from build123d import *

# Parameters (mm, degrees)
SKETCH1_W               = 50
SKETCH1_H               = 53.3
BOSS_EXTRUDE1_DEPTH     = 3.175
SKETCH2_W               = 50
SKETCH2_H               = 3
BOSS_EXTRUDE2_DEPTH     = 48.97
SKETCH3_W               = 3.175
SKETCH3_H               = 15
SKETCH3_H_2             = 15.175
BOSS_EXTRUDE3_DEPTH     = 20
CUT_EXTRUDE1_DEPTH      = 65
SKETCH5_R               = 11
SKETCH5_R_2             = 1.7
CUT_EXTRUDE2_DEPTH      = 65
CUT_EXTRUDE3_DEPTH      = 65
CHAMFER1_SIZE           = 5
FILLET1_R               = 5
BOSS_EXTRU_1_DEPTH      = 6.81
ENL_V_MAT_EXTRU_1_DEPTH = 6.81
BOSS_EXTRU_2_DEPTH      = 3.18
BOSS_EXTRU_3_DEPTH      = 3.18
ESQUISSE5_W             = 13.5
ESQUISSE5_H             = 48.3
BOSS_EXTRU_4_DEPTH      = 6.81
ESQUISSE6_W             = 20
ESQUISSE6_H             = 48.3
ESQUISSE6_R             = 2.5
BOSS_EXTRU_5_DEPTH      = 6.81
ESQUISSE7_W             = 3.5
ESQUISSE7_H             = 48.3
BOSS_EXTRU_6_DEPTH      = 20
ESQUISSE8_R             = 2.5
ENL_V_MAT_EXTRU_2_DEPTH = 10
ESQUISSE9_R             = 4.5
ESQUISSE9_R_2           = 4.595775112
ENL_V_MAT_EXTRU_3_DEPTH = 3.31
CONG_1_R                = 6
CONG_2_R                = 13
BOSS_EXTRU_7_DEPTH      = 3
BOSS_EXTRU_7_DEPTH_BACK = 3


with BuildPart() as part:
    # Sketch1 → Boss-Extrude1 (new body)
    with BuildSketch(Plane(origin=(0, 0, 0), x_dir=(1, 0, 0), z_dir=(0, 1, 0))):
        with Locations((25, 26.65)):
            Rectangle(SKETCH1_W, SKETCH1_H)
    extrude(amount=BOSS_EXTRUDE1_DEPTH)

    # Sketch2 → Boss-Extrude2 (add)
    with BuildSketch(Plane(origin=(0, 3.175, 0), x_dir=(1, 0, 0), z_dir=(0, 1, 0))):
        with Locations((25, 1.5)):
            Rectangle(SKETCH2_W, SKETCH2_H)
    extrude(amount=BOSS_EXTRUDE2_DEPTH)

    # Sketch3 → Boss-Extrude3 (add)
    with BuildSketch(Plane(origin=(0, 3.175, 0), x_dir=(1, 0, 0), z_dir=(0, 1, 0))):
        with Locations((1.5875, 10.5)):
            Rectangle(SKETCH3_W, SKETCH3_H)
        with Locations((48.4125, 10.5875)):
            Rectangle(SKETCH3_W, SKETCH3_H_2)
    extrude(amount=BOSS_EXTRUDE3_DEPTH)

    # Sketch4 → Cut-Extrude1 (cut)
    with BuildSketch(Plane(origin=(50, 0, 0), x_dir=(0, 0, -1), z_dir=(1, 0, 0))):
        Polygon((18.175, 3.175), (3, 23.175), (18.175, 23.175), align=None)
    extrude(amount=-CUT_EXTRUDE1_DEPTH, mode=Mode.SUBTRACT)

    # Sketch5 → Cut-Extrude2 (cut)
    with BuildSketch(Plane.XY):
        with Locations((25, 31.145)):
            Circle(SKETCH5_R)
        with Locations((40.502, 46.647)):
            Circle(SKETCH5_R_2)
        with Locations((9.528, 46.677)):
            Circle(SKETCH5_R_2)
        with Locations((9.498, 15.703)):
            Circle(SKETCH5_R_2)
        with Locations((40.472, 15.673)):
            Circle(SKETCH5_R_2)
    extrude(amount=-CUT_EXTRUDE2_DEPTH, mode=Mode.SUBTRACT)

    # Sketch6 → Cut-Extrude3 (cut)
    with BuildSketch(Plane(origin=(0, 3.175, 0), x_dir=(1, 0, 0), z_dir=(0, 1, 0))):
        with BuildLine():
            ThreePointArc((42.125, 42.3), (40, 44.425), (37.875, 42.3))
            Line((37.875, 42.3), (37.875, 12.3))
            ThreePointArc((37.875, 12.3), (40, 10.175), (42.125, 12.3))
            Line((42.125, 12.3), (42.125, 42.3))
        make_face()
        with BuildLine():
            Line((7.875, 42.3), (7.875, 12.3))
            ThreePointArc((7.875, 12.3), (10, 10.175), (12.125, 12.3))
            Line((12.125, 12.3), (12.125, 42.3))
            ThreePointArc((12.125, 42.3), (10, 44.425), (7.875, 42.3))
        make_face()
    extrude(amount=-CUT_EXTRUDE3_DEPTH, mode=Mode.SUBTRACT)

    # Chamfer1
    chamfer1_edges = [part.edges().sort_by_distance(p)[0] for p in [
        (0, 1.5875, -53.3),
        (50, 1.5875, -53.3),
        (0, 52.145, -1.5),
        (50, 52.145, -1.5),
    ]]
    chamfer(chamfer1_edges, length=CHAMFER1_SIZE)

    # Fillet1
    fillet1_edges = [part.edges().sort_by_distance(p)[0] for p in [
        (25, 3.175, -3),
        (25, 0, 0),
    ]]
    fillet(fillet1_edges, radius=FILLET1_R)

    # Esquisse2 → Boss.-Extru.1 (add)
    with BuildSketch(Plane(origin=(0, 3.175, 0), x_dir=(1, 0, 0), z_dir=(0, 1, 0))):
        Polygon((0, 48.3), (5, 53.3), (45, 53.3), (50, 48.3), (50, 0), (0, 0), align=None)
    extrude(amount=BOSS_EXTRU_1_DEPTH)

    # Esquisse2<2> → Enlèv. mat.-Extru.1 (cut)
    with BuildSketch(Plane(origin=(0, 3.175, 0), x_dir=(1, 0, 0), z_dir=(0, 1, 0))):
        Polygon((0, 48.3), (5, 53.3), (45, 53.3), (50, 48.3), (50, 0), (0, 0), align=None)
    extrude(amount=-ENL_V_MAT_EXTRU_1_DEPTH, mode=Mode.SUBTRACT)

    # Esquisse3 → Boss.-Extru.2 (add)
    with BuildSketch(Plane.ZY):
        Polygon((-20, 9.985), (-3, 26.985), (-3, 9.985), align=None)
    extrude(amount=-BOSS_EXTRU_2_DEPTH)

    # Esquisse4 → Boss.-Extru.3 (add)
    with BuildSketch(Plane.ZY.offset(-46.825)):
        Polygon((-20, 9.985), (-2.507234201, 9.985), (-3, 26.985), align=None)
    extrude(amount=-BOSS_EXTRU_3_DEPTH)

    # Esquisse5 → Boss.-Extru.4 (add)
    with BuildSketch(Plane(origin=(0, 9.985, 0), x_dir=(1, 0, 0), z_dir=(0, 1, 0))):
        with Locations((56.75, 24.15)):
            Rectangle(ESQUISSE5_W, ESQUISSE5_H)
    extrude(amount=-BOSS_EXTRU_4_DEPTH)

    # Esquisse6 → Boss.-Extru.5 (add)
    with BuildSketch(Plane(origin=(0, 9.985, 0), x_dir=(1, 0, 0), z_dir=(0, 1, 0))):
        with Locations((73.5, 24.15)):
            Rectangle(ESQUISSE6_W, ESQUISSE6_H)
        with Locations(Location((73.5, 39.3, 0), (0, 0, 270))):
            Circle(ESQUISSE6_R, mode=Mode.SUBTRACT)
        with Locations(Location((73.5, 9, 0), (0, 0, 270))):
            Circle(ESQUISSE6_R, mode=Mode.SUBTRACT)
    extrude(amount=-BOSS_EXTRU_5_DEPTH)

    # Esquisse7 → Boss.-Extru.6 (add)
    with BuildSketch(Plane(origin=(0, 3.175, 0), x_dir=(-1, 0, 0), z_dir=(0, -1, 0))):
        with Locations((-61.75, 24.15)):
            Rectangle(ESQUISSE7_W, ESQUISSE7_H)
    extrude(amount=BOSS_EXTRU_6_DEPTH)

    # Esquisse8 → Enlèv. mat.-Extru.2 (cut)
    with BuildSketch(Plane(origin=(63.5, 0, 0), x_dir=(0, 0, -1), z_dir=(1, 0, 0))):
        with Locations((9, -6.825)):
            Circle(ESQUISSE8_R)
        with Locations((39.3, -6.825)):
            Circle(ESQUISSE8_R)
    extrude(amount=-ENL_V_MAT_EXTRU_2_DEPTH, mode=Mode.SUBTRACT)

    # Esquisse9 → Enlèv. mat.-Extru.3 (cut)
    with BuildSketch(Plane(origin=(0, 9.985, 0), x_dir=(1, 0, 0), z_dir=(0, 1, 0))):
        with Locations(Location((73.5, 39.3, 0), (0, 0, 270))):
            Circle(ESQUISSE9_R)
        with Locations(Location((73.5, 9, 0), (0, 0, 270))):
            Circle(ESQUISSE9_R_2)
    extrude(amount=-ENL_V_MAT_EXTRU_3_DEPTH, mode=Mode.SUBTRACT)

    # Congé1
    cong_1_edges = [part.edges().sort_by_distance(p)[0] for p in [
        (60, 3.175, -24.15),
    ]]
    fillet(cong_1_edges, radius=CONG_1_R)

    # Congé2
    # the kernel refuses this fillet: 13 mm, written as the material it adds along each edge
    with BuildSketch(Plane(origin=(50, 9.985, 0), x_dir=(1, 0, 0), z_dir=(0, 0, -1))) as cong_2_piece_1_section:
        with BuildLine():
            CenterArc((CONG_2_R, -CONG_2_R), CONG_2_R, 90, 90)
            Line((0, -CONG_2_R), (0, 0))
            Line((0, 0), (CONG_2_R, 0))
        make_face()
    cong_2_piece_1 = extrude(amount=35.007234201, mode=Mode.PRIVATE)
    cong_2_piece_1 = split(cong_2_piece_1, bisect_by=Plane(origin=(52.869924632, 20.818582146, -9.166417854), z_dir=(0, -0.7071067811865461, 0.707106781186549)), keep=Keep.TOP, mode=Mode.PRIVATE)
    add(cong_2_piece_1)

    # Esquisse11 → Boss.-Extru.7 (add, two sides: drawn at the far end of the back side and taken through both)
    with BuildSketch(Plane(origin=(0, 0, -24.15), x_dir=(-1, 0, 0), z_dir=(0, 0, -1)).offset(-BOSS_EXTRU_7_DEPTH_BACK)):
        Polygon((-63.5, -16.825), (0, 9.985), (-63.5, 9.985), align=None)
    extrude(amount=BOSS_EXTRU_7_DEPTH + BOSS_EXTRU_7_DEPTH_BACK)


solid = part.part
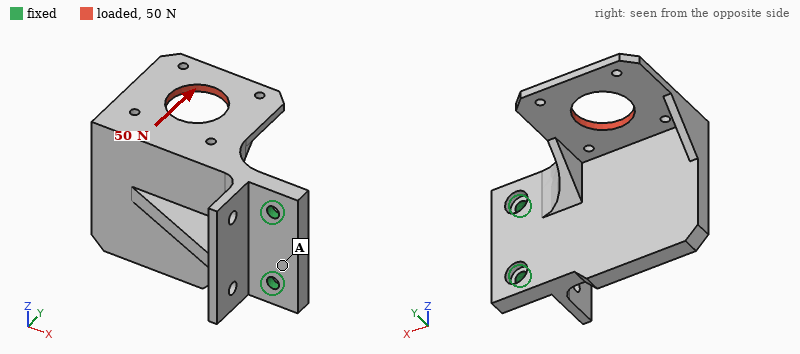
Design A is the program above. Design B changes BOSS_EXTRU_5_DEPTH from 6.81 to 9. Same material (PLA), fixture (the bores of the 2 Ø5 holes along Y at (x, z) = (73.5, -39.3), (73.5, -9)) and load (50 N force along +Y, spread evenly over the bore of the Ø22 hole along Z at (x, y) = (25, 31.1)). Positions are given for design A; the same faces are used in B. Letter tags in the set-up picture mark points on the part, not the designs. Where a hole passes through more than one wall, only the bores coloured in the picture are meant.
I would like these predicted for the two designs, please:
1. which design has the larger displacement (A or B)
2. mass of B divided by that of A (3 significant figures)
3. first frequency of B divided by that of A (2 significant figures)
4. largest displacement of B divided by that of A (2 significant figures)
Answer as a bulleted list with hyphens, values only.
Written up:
- A
- 1.05
- 1.5
- 0.53
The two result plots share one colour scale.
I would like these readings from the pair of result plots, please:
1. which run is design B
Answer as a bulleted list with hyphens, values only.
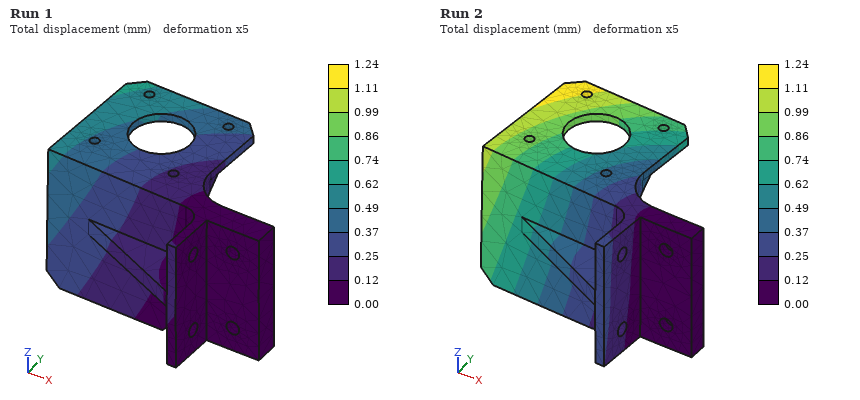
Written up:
- Run 1
